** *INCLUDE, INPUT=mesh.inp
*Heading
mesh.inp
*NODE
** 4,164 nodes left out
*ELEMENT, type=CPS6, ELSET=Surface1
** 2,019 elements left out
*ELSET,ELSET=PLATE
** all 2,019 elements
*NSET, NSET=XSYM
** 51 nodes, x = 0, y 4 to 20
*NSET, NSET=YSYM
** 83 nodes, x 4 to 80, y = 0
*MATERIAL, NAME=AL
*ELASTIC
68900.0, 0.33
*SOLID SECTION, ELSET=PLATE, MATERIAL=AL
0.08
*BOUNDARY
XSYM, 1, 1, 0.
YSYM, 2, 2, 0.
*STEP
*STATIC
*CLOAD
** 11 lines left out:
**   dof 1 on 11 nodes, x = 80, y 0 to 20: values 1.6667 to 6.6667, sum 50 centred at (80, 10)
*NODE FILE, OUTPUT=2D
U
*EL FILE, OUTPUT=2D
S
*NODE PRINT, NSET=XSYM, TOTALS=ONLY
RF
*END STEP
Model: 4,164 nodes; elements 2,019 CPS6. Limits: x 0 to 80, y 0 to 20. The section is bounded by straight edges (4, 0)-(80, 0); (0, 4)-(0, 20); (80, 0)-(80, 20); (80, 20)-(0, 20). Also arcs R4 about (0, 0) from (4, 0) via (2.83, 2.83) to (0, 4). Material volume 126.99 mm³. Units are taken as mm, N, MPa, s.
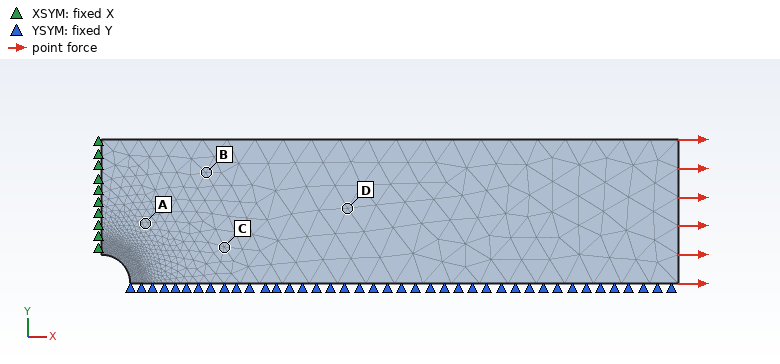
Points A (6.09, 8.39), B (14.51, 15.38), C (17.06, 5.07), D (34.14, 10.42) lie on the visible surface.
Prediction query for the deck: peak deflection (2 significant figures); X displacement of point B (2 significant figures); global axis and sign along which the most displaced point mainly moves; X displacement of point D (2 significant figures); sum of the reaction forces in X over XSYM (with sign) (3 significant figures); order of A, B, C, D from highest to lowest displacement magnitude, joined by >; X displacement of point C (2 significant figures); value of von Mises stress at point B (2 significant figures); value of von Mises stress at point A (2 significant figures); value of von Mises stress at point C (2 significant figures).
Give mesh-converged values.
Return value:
0.038 mm
0.0071 mm
+X
0.016 mm
-50.0 N
D > C > B > A
0.0090 mm
34 MPa
39 MPa
29 MPa
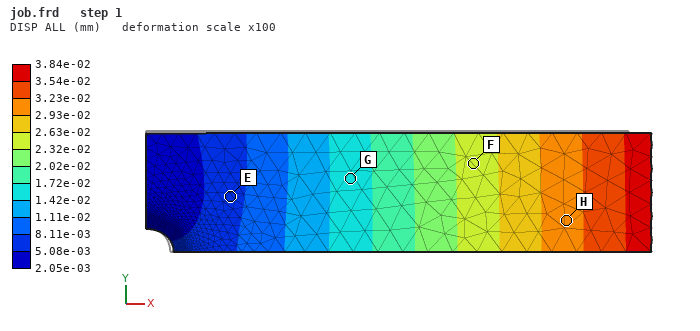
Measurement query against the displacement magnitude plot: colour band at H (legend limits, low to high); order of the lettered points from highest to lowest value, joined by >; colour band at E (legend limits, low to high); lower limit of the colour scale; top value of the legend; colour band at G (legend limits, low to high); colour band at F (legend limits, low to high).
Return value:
2.93e-02 to 3.23e-02 mm
H > F > G > E
5.08e-03 to 8.11e-03 mm
2.05e-03 mm
3.84e-02 mm
1.42e-02 to 1.72e-02 mm
2.32e-02 to 2.63e-02 mm
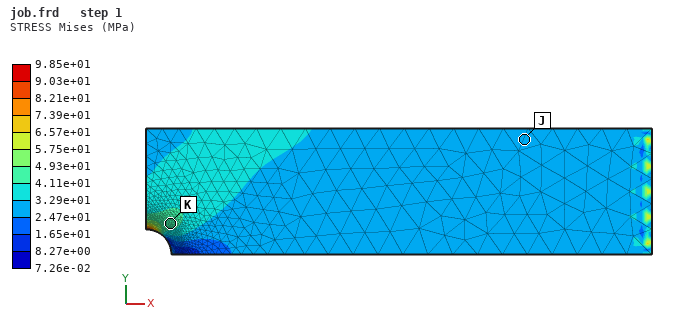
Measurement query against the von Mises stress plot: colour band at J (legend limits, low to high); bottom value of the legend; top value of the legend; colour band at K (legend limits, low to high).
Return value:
2.47e+01 to 3.29e+01 MPa
7.26e-02 MPa
9.85e+01 MPa
4.11e+01 to 4.93e+01 MPa
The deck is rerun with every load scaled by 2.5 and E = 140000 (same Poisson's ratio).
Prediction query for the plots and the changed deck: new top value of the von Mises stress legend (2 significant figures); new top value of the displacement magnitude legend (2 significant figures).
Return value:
250 MPa
0.047 mm
